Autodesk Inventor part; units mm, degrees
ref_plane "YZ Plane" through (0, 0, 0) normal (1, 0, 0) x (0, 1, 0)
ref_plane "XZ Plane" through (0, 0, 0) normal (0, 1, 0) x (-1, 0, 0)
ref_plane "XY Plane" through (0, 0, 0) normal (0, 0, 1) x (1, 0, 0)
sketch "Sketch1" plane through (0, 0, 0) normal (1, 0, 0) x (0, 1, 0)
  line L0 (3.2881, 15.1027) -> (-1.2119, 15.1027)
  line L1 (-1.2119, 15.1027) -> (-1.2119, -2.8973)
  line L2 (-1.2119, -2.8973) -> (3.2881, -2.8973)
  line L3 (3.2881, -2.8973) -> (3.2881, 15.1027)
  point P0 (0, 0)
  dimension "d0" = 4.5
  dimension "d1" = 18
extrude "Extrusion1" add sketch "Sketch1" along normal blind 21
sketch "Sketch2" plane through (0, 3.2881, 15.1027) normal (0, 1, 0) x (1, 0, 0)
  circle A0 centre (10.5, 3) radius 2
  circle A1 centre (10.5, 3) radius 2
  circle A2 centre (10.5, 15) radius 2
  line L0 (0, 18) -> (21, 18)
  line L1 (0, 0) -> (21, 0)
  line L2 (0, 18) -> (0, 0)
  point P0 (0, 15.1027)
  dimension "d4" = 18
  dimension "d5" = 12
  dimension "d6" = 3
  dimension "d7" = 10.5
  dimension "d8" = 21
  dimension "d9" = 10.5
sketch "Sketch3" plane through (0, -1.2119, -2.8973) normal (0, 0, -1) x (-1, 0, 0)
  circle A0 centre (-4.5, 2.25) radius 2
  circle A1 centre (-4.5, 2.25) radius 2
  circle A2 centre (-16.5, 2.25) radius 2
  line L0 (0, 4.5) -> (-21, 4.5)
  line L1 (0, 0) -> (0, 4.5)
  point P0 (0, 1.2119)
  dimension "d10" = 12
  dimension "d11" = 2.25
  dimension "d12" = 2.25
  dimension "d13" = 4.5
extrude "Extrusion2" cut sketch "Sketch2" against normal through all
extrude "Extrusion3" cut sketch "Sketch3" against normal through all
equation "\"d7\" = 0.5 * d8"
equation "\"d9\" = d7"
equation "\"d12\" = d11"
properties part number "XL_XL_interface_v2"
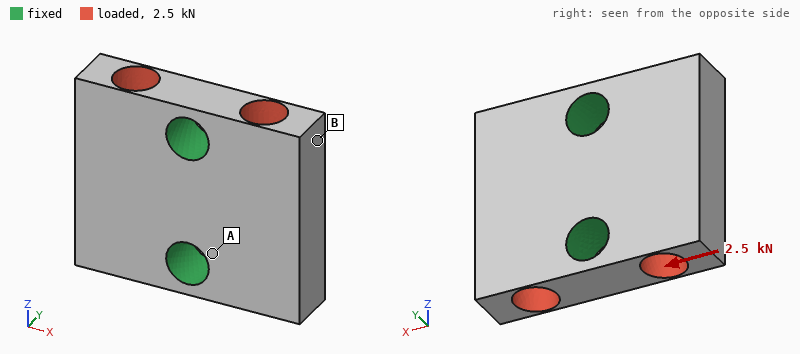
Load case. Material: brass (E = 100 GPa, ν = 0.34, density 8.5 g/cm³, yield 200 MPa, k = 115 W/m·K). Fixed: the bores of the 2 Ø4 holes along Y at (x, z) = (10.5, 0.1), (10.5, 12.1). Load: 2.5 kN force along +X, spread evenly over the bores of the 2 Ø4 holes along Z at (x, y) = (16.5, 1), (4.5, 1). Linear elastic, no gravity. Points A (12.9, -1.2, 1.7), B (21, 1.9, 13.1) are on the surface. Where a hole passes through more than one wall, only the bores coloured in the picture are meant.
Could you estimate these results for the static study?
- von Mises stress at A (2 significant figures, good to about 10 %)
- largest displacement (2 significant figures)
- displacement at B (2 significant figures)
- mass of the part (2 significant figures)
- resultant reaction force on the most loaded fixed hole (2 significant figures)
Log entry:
36 MPa
3.6 µm
3.3 µm
9.7 g
1.3 kN
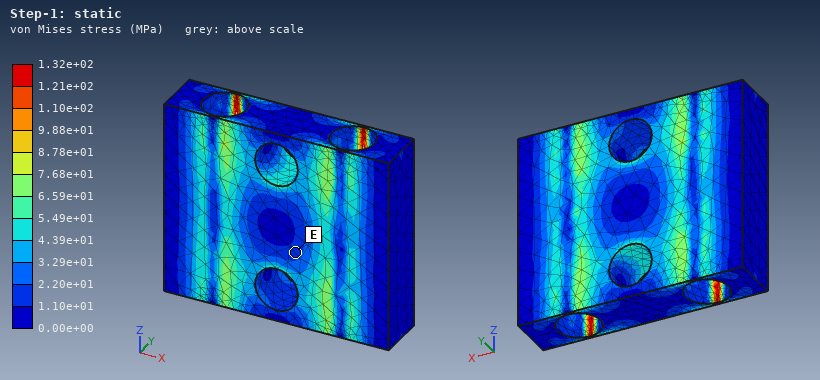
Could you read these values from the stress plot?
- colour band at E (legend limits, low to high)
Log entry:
1.10e+01 to 2.20e+01 MPa
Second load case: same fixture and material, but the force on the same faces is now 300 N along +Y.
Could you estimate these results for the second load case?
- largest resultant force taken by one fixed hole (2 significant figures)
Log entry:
150 N
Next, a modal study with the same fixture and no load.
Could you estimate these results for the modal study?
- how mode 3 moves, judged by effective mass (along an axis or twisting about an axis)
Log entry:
twisting about X
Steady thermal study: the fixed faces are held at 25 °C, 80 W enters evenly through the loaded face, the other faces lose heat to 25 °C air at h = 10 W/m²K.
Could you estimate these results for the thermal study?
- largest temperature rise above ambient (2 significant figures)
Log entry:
61 K
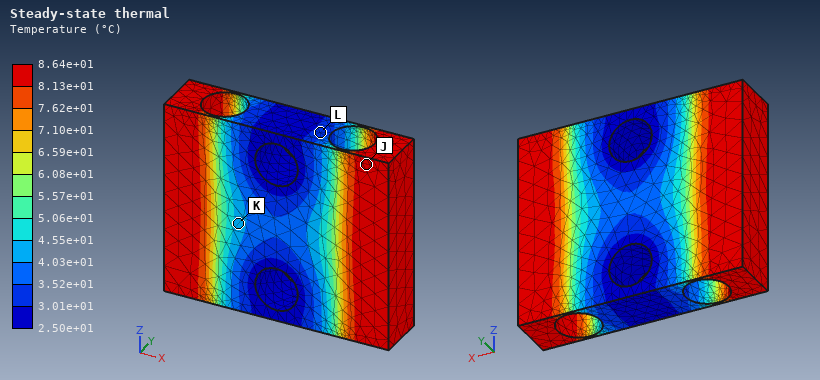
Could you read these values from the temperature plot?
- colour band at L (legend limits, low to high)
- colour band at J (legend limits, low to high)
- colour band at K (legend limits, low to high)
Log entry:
3.01e+01 to 3.52e+01 °C
8.13e+01 to 8.64e+01 °C
4.03e+01 to 4.55e+01 °C
